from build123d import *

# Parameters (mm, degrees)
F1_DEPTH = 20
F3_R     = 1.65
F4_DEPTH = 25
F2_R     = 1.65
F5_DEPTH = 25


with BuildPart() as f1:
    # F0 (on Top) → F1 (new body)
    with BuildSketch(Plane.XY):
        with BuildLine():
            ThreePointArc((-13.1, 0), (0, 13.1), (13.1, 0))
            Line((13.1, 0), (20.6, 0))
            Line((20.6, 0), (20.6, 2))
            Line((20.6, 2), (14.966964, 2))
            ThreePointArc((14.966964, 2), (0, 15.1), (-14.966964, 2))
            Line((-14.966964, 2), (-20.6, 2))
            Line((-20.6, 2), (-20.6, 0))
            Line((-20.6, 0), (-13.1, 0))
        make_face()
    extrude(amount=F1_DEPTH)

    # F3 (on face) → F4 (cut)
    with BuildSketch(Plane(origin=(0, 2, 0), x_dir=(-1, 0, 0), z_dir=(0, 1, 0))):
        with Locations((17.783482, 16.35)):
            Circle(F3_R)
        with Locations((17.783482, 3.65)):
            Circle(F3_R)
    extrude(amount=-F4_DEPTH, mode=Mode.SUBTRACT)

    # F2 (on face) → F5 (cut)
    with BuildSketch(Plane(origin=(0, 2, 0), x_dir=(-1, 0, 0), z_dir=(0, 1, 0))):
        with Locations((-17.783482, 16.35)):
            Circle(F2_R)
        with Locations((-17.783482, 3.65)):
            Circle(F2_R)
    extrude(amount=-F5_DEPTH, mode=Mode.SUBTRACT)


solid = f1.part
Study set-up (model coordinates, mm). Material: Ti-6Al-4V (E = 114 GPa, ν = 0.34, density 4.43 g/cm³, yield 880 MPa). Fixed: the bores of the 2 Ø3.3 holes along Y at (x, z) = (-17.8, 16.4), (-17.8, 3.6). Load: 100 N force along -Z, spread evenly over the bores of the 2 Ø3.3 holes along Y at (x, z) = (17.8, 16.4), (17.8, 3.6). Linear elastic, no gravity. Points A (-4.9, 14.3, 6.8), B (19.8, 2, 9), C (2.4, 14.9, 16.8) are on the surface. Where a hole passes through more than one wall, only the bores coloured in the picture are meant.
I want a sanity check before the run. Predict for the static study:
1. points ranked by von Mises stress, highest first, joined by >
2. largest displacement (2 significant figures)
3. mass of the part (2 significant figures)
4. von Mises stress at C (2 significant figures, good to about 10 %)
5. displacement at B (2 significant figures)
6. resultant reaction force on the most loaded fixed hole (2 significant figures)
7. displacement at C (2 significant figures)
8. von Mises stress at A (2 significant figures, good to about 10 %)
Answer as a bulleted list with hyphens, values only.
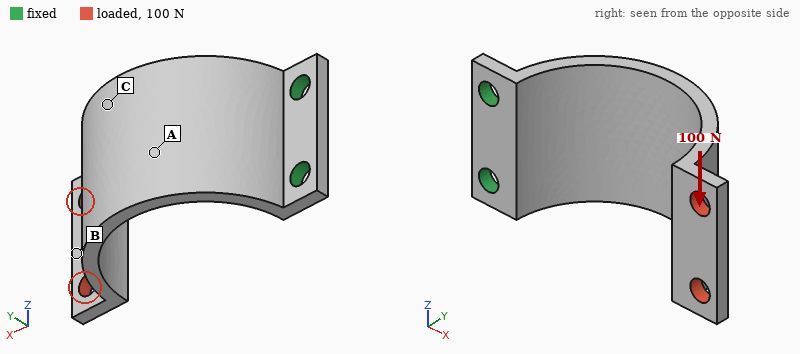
- A > C > B
- 0.57 mm
- 9.5 g
- 73 MPa
- 0.49 mm
- 240 N
- 0.16 mm
- 120 MPa
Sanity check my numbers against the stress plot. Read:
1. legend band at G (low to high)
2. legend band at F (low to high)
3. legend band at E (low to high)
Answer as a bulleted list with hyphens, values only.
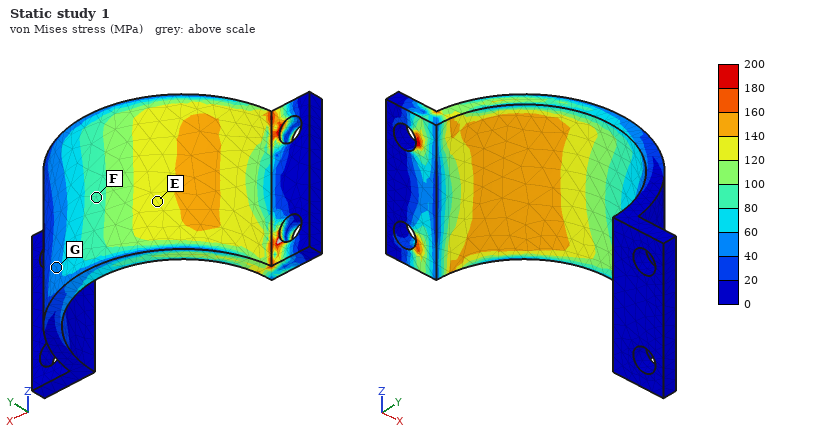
- 40 to 60 MPa
- 80 to 100 MPa
- 120 to 140 MPa
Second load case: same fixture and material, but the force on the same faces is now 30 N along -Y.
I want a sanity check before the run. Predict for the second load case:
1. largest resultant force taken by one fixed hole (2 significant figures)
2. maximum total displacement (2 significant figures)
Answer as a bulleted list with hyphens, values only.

- 17 N
- 0.44 mm
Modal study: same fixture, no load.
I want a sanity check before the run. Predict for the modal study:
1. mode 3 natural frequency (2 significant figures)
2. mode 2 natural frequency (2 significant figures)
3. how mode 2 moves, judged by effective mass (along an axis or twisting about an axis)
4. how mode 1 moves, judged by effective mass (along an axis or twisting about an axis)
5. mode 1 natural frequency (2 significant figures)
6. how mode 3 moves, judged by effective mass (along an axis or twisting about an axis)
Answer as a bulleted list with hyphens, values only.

- 2600 Hz
- 1400 Hz
- along Z
- along Y
- 830 Hz
- along X
